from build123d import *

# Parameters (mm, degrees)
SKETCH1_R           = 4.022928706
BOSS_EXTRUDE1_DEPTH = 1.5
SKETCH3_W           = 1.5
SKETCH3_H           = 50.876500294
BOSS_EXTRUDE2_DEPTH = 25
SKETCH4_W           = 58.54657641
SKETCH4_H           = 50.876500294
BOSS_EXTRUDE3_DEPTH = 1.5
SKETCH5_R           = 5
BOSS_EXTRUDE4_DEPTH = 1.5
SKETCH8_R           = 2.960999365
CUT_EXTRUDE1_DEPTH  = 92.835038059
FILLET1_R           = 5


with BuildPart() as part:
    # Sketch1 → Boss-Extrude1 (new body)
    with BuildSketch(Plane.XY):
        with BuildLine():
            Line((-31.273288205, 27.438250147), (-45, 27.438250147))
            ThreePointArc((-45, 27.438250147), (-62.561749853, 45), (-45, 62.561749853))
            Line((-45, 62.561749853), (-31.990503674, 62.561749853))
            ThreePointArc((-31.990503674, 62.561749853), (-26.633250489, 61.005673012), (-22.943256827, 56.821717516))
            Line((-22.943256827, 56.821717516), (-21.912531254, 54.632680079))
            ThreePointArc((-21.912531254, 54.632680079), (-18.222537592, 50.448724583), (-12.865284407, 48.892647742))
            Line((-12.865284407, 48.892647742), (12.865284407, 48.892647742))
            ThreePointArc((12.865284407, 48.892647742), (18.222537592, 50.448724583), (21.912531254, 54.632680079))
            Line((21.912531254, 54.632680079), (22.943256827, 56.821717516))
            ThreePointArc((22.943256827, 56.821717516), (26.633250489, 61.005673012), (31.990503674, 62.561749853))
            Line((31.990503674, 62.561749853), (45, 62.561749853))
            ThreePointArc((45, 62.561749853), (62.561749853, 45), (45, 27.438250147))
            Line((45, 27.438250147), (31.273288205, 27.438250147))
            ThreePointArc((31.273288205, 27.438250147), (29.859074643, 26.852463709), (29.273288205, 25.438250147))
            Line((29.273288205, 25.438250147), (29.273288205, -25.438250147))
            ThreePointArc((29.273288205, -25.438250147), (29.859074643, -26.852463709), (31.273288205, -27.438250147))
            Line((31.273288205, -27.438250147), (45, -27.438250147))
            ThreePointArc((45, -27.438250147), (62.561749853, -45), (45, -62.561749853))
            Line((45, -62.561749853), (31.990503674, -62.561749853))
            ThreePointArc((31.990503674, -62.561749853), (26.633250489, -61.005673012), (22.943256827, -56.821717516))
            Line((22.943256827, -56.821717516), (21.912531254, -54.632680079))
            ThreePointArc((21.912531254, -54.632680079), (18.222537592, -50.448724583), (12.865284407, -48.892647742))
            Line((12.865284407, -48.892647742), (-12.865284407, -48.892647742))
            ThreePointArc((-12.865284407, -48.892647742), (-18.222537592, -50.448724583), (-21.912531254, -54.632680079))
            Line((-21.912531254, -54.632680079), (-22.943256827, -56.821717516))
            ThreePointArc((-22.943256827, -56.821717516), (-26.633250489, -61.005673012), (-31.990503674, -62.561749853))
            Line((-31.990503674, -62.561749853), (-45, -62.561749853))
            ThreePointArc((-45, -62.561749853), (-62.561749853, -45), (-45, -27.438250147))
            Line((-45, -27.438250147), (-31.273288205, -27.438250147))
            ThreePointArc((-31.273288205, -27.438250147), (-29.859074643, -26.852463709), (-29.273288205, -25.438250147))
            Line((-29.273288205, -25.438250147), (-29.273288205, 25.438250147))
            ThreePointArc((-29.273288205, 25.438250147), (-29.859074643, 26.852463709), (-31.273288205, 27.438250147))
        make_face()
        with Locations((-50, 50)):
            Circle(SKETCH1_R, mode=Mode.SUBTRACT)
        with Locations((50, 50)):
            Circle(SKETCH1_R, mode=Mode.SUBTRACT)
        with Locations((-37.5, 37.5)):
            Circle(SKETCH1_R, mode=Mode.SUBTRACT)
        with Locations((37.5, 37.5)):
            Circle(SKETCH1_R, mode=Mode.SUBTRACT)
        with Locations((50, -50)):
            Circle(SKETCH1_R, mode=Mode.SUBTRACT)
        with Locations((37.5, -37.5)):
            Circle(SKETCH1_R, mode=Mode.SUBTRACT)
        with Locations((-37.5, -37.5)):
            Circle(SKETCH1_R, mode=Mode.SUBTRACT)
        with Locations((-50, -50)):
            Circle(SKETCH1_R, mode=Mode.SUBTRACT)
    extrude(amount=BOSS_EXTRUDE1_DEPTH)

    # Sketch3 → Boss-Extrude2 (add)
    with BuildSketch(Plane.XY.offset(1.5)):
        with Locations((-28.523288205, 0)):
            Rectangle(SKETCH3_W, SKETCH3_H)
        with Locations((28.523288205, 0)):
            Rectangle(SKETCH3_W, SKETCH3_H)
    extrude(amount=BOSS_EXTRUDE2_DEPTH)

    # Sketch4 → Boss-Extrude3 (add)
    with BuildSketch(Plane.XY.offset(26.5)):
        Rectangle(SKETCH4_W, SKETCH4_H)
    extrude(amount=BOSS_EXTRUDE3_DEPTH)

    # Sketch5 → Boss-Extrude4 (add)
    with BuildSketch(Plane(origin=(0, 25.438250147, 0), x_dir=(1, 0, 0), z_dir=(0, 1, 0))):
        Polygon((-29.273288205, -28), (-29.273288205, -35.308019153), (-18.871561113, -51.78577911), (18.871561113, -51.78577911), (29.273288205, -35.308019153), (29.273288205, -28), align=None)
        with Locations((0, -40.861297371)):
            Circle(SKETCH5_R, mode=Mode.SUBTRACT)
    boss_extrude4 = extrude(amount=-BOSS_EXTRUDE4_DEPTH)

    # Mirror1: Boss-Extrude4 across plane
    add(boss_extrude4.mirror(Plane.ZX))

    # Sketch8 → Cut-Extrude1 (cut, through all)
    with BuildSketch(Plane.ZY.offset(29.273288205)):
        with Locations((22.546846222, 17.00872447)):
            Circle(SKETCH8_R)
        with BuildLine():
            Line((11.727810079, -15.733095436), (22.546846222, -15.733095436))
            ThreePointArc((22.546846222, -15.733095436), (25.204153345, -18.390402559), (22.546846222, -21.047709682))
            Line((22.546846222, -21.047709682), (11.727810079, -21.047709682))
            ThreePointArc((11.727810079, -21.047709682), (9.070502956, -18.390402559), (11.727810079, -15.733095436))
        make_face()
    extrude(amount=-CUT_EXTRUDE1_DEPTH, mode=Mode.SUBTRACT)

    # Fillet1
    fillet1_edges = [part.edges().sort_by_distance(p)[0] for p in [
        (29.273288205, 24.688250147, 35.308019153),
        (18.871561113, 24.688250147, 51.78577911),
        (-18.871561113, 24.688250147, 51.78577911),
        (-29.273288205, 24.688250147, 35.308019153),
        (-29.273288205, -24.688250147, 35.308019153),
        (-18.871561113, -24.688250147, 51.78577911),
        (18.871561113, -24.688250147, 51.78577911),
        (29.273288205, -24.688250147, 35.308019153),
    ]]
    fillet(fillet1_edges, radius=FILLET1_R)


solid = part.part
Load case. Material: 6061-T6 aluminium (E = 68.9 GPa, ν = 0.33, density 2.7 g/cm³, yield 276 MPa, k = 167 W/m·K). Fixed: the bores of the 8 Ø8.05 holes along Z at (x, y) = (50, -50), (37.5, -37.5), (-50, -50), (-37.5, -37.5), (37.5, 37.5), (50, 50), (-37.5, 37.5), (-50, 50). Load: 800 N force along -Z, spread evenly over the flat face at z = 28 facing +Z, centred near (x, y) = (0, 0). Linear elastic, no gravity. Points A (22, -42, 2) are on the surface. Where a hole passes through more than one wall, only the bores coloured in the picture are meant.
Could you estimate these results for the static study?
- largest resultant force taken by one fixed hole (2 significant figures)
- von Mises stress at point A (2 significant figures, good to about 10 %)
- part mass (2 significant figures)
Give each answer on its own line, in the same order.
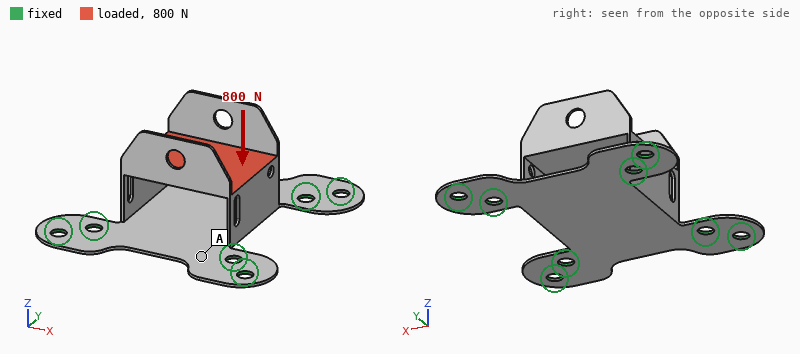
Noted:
230 N
30 MPa
71 g
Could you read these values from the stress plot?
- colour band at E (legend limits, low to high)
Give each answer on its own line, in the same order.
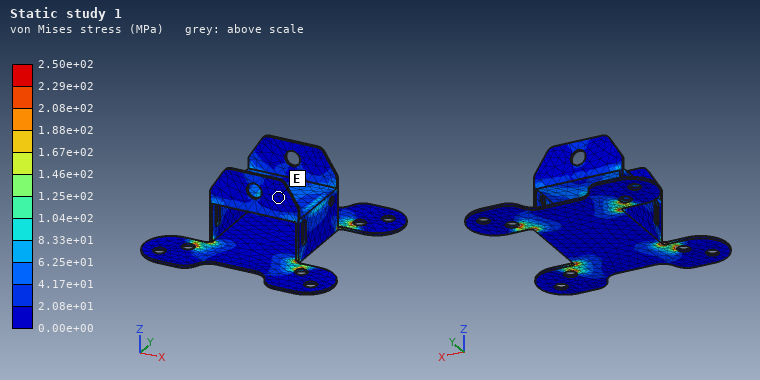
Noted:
0.00e+00 to 2.08e+01 MPa
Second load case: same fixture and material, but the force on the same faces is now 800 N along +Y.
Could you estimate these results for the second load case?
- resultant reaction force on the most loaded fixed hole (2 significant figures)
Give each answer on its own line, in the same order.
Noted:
290 N
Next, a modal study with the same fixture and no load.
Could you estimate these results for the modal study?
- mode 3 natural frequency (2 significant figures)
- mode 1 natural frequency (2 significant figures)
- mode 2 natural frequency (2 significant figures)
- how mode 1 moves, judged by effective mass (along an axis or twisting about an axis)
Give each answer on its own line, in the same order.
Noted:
1300 Hz
740 Hz
1300 Hz
along X
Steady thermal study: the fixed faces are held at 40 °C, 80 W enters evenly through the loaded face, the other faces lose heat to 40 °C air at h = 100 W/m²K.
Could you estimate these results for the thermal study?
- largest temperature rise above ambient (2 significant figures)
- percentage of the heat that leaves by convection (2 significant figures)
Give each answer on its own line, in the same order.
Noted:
71 K
87 %
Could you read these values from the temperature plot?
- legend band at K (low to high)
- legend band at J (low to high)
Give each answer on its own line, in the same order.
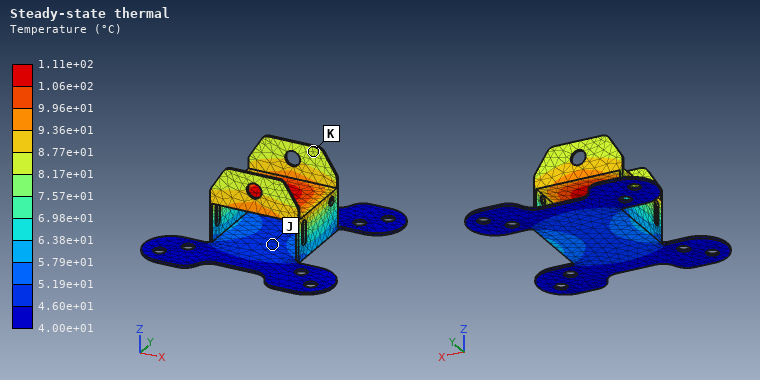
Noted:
8.17e+01 to 8.77e+01 °C
4.60e+01 to 5.19e+01 °C
